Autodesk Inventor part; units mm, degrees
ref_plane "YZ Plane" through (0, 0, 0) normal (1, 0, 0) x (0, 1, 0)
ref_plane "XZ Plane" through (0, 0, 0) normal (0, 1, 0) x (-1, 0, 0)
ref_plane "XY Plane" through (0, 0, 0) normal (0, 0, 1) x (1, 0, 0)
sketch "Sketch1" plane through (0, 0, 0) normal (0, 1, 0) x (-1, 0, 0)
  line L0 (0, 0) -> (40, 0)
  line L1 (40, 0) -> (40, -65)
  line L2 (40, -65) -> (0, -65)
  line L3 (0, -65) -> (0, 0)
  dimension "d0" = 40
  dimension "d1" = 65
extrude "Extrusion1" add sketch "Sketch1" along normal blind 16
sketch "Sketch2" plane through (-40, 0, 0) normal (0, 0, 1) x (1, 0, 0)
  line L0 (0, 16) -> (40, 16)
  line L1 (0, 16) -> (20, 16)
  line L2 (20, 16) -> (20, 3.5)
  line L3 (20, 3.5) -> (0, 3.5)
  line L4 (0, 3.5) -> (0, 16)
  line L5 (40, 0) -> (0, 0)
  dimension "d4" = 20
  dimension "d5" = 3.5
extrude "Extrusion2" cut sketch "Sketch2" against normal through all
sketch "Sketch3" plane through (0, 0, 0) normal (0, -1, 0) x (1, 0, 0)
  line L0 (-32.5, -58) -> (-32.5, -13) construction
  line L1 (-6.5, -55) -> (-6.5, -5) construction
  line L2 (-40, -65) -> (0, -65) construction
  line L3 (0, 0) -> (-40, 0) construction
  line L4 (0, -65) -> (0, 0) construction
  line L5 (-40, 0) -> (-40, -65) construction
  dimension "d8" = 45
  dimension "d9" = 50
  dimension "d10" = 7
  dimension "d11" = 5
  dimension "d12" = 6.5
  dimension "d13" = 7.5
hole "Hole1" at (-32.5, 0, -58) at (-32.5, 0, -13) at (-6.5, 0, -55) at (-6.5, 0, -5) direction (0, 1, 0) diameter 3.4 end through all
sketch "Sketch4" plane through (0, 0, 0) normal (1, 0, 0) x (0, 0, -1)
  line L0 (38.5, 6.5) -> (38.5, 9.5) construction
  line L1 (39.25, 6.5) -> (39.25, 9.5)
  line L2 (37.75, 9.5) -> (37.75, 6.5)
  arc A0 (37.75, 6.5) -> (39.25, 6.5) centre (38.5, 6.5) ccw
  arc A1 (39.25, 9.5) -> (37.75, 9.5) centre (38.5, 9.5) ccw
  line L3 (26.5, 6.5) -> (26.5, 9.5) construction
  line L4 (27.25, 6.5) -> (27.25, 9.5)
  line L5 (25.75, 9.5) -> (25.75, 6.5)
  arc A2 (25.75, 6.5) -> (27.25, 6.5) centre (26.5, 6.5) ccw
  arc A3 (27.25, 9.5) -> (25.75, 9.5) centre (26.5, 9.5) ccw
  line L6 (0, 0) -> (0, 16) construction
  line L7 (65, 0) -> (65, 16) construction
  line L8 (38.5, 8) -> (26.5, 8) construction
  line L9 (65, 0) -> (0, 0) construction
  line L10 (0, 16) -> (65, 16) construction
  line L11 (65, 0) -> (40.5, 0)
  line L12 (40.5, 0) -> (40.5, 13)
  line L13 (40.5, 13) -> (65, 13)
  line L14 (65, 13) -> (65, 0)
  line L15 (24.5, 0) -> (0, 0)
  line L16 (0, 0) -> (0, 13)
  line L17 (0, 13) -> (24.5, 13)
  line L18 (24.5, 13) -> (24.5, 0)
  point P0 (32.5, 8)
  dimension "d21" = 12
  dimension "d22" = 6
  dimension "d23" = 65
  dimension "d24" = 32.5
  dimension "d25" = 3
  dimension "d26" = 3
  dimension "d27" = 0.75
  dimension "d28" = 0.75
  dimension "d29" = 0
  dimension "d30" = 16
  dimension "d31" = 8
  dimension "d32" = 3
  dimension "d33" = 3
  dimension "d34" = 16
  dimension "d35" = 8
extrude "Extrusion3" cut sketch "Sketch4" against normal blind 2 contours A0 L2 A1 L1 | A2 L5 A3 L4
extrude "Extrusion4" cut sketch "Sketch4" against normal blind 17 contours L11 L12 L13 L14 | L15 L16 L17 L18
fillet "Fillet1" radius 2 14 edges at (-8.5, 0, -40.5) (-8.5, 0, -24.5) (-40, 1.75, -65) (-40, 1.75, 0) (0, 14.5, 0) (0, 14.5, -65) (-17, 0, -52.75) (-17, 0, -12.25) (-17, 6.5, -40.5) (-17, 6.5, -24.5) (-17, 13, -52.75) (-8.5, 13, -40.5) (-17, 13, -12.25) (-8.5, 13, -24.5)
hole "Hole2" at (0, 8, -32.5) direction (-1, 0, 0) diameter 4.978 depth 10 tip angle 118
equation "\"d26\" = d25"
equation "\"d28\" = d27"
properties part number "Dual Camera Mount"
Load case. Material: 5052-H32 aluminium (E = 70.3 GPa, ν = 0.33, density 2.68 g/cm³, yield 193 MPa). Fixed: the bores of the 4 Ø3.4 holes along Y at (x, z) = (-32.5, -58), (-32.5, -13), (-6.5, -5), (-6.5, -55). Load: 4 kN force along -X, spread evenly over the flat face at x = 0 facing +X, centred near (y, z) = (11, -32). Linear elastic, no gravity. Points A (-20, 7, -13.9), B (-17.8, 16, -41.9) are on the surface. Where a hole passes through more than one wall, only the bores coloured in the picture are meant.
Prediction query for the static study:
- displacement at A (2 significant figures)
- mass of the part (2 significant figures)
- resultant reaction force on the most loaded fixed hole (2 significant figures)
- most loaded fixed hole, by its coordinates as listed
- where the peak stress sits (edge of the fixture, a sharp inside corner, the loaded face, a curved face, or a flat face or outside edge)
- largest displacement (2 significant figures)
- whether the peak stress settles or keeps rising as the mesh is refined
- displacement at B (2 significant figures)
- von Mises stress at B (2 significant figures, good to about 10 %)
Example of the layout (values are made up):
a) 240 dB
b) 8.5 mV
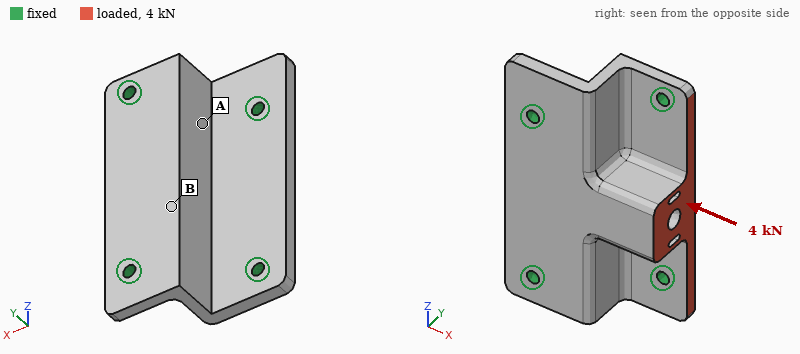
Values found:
a) 5.7 µm
b) 38 g
c) 1.5 kN
d) (-6.5, -55)
e) edge of the fixture
f) 28 µm
g) keeps rising
h) 17 µm
i) 31 MPa
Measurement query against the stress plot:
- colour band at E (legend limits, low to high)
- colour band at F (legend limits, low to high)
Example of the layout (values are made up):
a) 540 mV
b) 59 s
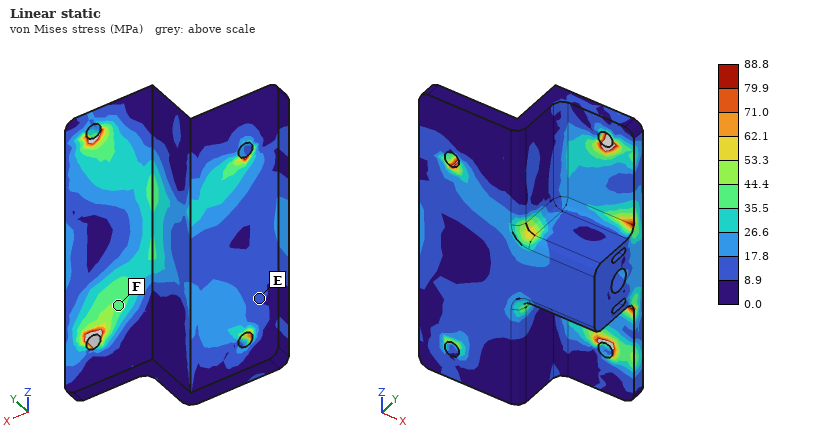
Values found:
a) 8.9 to 17.8 MPa
b) 35.5 to 44.4 MPa
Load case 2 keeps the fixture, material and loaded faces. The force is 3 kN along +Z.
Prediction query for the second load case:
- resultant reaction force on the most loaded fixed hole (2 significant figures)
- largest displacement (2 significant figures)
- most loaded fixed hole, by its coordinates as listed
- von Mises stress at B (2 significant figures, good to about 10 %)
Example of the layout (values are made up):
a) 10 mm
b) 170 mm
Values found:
a) 1.4 kN
b) 23 µm
c) (-6.5, -55)
d) 12 MPa
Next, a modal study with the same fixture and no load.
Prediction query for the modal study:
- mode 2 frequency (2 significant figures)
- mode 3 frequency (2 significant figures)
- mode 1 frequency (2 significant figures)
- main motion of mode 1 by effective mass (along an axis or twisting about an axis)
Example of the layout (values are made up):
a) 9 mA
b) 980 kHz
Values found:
a) 11 kHz
b) 14 kHz
c) 6700 Hz
d) along Y
